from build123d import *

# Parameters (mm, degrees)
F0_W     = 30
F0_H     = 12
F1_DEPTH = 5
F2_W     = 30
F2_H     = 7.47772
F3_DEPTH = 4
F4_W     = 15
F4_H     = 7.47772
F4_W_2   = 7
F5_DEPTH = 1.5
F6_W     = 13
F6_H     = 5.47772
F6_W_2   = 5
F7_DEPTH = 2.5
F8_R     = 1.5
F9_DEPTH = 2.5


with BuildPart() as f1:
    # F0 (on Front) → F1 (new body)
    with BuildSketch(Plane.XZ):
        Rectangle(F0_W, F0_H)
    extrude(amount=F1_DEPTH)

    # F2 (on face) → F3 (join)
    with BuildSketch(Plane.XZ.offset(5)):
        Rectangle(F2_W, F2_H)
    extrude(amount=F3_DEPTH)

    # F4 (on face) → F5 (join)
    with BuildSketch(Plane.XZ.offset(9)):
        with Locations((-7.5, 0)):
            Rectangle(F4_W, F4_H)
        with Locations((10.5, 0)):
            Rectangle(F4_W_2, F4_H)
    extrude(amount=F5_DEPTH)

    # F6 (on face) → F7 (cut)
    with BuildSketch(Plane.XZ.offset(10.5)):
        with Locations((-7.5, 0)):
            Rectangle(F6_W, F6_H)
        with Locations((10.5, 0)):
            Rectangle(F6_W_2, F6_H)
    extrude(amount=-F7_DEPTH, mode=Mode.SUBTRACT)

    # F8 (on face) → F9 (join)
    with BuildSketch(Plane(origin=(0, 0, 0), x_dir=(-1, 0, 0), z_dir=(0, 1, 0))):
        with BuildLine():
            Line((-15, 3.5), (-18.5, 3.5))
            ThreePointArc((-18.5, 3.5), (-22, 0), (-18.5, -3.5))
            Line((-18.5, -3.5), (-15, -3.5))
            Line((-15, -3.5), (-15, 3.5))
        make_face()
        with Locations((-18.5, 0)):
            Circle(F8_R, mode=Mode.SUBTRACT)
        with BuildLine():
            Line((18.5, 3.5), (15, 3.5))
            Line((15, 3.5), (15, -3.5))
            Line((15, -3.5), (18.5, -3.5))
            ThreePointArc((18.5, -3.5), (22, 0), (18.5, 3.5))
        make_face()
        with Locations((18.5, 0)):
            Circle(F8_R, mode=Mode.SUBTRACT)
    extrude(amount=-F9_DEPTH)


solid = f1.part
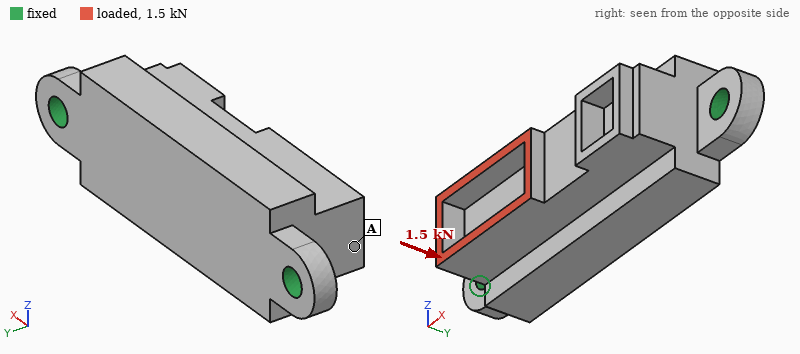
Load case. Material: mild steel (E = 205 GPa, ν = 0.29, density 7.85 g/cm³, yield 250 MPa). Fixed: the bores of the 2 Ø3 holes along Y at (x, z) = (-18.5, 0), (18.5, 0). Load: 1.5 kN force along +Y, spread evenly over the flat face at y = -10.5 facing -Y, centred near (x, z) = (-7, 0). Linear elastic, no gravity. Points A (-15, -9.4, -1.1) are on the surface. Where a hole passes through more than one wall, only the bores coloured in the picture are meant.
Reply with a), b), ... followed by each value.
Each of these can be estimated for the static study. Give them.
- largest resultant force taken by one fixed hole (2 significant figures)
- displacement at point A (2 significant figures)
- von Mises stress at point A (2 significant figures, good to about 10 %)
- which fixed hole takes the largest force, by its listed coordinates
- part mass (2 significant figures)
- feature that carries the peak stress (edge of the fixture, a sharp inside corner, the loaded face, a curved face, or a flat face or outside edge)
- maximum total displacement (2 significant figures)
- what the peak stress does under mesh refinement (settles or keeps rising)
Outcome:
a) 1.2 kN
b) 7.4 µm
c) 37 MPa
d) (-18.5, 0)
e) 23 g
f) edge of the fixture
g) 9.7 µm
h) keeps rising
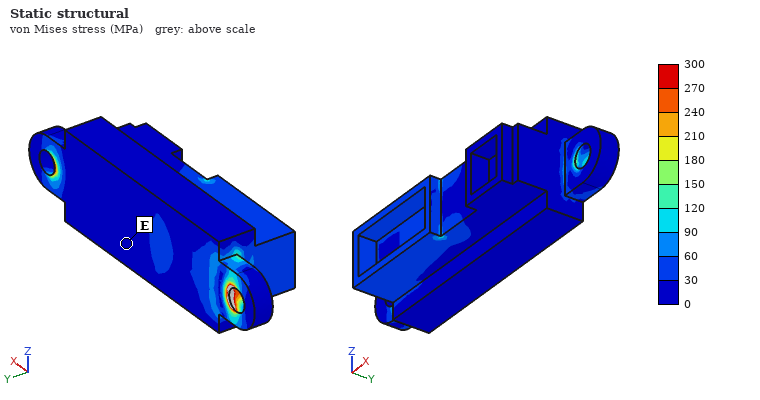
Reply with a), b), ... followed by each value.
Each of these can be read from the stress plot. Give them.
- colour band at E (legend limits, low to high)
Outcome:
a) 0 to 30 MPa
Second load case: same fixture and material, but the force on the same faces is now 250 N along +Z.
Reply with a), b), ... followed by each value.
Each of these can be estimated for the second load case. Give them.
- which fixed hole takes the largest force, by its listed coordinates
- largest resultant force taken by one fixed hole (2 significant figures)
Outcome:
a) (-18.5, 0)
b) 180 N
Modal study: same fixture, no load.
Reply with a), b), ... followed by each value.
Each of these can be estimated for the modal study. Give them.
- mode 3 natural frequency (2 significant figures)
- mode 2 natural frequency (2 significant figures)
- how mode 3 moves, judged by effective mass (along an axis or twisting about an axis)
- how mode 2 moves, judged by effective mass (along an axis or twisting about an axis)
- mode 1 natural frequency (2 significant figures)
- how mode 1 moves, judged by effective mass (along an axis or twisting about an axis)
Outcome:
a) 21 kHz
b) 15 kHz
c) along Z
d) along Y
e) 8900 Hz
f) along Z
